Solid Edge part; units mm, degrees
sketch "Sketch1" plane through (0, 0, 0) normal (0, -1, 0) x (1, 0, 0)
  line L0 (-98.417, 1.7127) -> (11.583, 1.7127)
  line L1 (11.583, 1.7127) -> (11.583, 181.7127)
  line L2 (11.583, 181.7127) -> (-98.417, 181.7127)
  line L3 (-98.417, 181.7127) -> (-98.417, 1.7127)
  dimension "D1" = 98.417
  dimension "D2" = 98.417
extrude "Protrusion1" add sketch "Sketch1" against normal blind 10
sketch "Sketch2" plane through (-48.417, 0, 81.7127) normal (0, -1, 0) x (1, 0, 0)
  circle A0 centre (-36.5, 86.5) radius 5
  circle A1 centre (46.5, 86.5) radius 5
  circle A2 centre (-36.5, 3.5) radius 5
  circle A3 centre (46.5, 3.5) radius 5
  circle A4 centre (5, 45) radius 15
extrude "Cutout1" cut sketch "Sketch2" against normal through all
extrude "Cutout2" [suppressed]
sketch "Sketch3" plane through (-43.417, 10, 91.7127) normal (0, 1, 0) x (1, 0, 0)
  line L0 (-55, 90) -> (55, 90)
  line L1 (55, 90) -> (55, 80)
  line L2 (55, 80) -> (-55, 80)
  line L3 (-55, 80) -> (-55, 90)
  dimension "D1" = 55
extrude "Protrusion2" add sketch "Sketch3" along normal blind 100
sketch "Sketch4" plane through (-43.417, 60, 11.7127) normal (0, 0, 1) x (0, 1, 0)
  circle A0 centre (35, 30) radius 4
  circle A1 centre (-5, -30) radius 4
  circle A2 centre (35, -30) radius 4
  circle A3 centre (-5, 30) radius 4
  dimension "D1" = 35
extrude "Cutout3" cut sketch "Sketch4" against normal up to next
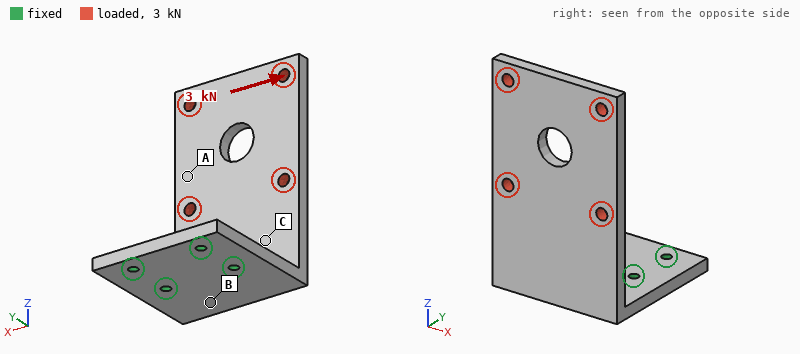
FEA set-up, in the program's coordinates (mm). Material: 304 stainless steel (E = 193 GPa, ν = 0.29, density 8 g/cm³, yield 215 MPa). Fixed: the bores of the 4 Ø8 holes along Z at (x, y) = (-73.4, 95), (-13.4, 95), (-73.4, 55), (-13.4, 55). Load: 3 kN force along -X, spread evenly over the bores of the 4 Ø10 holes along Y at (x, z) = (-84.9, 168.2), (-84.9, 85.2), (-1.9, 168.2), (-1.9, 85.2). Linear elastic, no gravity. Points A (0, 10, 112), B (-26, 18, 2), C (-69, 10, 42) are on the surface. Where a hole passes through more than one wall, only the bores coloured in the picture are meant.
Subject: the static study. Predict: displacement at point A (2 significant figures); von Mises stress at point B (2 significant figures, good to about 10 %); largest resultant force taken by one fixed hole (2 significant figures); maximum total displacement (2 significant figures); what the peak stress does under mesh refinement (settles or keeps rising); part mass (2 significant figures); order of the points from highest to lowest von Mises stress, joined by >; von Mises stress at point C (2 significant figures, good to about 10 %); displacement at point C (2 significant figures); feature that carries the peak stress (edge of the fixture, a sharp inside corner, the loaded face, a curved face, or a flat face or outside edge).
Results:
0.34 mm
80 MPa
6.2 kN
0.55 mm
keeps rising
2.4 kg
B > C > A
31 MPa
0.13 mm
edge of the fixture
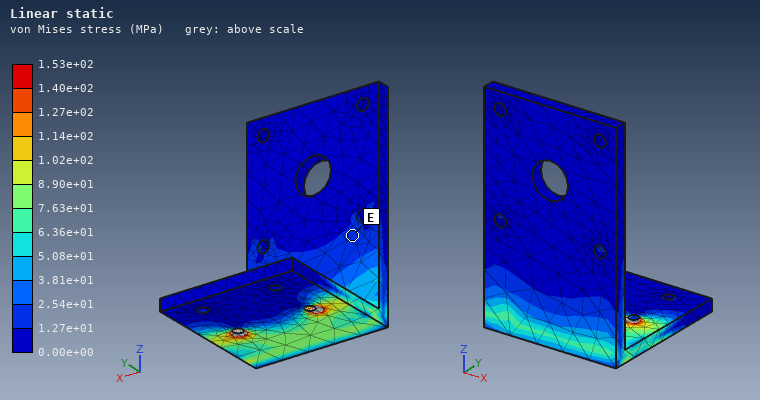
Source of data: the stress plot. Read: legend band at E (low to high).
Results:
1.27e+01 to 2.54e+01 MPa
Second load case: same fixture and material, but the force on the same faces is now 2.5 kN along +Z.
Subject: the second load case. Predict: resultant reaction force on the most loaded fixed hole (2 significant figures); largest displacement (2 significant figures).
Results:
1.8 kN
0.33 mm
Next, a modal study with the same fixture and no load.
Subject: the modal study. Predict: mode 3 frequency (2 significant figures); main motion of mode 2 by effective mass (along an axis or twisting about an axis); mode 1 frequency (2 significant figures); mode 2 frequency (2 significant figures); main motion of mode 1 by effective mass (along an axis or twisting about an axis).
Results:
870 Hz
along X
190 Hz
440 Hz
along Y
